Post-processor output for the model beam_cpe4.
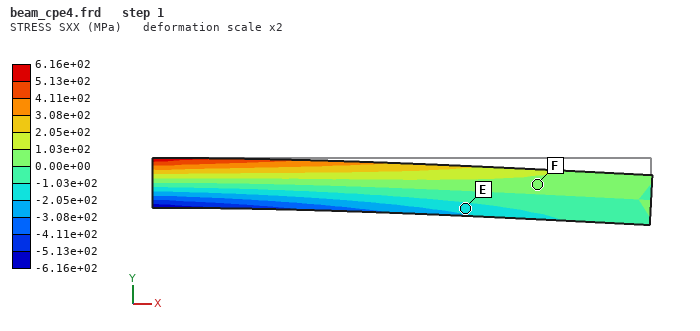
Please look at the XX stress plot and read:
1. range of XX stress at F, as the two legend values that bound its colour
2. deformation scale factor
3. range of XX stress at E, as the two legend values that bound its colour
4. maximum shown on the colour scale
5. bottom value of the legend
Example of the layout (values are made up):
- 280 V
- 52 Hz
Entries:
- 0.00e+00 to 1.03e+02 MPa
- 2
- -2.05e+02 to -1.03e+02 MPa
- 6.16e+02 MPa
- -6.16e+02 MPa
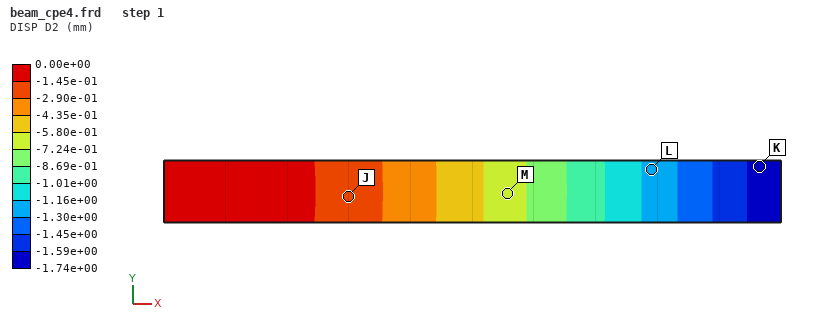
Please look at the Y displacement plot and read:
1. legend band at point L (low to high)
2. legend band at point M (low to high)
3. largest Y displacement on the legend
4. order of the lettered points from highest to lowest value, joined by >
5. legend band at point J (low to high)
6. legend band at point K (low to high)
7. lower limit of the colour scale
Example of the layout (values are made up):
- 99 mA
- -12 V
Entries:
- -1.30e+00 to -1.16e+00 mm
- -7.24e-01 to -5.80e-01 mm
- 0.00e+00 mm
- J > M > L > K
- -2.90e-01 to -1.45e-01 mm
- -1.74e+00 to -1.59e+00 mm
- -1.74e+00 mm
